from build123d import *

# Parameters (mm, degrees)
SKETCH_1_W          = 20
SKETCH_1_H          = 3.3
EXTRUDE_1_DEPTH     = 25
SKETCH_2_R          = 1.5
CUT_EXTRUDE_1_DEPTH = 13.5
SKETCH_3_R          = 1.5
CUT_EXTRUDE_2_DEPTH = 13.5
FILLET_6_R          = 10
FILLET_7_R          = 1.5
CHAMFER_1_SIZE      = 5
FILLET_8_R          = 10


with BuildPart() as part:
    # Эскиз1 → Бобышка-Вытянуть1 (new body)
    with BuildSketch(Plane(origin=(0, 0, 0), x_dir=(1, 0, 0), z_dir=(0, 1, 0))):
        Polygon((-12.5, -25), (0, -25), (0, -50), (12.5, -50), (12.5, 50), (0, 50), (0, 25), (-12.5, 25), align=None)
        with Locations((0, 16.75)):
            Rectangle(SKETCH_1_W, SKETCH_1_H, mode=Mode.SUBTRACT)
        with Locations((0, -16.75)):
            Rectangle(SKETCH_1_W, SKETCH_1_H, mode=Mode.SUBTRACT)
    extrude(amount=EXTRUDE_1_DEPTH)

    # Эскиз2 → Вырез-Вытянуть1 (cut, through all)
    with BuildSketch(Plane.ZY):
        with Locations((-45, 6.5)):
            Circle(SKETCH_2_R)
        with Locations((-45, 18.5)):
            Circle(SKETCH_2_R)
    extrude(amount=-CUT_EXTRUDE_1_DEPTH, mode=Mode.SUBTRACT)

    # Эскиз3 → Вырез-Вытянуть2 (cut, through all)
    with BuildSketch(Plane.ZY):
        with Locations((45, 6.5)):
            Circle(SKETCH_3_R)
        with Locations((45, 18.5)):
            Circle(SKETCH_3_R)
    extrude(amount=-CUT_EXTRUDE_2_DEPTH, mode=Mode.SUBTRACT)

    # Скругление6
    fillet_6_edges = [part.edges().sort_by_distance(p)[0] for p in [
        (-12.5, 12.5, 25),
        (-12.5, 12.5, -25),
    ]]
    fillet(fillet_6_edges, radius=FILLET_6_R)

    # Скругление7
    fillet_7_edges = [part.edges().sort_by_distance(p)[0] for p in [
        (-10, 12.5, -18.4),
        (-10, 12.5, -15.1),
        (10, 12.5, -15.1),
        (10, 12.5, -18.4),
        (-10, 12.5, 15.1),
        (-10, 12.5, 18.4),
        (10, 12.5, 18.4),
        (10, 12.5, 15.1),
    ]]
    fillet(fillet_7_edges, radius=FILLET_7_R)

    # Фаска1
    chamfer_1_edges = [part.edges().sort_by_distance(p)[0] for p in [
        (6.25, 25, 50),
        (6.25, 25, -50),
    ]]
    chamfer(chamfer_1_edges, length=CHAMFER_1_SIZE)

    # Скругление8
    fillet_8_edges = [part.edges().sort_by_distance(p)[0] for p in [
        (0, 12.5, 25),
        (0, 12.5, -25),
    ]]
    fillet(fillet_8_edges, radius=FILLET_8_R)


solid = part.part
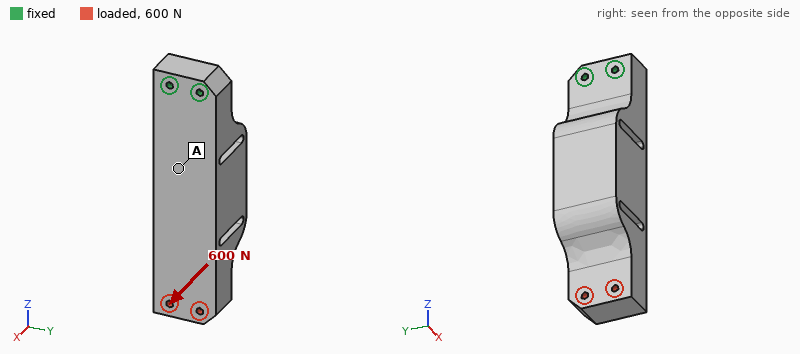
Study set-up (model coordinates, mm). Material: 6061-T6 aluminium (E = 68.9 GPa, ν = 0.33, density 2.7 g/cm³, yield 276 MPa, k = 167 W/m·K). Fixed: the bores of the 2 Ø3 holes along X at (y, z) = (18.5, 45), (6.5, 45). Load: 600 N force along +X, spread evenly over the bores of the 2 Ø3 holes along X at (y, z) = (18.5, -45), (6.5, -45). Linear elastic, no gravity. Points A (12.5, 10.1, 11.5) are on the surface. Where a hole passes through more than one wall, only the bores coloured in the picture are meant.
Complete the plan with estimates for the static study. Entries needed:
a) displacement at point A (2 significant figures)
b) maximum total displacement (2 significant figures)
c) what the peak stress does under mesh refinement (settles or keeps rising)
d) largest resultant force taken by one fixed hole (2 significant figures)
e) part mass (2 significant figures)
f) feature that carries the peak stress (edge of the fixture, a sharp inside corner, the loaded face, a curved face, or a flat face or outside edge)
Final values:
0.11 mm
0.43 mm
keeps rising
320 N
110 g
edge of the fixture
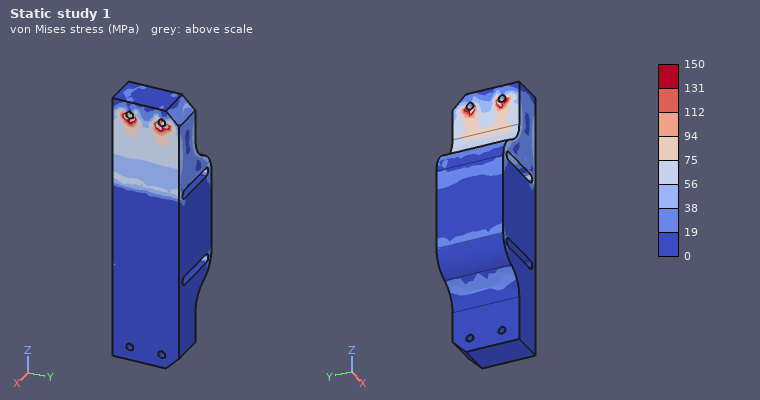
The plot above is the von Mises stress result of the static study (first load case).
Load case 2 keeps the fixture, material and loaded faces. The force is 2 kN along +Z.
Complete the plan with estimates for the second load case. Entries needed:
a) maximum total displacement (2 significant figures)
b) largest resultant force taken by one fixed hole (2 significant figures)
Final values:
16 µm
1.0 kN
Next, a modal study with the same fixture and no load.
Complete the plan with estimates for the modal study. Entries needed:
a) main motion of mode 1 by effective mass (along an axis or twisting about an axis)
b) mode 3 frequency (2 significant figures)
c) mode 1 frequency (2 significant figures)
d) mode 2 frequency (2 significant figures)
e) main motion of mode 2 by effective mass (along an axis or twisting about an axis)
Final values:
along X
5100 Hz
1100 Hz
1600 Hz
along Y
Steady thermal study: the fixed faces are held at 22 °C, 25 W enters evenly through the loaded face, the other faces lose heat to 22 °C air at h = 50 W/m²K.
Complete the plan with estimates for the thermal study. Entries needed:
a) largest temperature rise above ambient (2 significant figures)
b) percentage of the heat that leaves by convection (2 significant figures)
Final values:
37 K
38 %
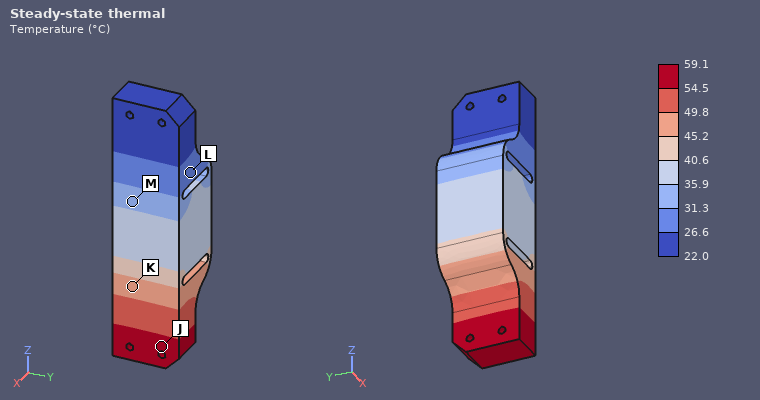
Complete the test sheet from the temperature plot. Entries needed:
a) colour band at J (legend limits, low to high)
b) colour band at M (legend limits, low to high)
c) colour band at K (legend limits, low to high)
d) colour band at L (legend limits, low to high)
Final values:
54.5 to 59.1 °C
31.3 to 35.9 °C
45.2 to 49.8 °C
26.6 to 31.3 °C
